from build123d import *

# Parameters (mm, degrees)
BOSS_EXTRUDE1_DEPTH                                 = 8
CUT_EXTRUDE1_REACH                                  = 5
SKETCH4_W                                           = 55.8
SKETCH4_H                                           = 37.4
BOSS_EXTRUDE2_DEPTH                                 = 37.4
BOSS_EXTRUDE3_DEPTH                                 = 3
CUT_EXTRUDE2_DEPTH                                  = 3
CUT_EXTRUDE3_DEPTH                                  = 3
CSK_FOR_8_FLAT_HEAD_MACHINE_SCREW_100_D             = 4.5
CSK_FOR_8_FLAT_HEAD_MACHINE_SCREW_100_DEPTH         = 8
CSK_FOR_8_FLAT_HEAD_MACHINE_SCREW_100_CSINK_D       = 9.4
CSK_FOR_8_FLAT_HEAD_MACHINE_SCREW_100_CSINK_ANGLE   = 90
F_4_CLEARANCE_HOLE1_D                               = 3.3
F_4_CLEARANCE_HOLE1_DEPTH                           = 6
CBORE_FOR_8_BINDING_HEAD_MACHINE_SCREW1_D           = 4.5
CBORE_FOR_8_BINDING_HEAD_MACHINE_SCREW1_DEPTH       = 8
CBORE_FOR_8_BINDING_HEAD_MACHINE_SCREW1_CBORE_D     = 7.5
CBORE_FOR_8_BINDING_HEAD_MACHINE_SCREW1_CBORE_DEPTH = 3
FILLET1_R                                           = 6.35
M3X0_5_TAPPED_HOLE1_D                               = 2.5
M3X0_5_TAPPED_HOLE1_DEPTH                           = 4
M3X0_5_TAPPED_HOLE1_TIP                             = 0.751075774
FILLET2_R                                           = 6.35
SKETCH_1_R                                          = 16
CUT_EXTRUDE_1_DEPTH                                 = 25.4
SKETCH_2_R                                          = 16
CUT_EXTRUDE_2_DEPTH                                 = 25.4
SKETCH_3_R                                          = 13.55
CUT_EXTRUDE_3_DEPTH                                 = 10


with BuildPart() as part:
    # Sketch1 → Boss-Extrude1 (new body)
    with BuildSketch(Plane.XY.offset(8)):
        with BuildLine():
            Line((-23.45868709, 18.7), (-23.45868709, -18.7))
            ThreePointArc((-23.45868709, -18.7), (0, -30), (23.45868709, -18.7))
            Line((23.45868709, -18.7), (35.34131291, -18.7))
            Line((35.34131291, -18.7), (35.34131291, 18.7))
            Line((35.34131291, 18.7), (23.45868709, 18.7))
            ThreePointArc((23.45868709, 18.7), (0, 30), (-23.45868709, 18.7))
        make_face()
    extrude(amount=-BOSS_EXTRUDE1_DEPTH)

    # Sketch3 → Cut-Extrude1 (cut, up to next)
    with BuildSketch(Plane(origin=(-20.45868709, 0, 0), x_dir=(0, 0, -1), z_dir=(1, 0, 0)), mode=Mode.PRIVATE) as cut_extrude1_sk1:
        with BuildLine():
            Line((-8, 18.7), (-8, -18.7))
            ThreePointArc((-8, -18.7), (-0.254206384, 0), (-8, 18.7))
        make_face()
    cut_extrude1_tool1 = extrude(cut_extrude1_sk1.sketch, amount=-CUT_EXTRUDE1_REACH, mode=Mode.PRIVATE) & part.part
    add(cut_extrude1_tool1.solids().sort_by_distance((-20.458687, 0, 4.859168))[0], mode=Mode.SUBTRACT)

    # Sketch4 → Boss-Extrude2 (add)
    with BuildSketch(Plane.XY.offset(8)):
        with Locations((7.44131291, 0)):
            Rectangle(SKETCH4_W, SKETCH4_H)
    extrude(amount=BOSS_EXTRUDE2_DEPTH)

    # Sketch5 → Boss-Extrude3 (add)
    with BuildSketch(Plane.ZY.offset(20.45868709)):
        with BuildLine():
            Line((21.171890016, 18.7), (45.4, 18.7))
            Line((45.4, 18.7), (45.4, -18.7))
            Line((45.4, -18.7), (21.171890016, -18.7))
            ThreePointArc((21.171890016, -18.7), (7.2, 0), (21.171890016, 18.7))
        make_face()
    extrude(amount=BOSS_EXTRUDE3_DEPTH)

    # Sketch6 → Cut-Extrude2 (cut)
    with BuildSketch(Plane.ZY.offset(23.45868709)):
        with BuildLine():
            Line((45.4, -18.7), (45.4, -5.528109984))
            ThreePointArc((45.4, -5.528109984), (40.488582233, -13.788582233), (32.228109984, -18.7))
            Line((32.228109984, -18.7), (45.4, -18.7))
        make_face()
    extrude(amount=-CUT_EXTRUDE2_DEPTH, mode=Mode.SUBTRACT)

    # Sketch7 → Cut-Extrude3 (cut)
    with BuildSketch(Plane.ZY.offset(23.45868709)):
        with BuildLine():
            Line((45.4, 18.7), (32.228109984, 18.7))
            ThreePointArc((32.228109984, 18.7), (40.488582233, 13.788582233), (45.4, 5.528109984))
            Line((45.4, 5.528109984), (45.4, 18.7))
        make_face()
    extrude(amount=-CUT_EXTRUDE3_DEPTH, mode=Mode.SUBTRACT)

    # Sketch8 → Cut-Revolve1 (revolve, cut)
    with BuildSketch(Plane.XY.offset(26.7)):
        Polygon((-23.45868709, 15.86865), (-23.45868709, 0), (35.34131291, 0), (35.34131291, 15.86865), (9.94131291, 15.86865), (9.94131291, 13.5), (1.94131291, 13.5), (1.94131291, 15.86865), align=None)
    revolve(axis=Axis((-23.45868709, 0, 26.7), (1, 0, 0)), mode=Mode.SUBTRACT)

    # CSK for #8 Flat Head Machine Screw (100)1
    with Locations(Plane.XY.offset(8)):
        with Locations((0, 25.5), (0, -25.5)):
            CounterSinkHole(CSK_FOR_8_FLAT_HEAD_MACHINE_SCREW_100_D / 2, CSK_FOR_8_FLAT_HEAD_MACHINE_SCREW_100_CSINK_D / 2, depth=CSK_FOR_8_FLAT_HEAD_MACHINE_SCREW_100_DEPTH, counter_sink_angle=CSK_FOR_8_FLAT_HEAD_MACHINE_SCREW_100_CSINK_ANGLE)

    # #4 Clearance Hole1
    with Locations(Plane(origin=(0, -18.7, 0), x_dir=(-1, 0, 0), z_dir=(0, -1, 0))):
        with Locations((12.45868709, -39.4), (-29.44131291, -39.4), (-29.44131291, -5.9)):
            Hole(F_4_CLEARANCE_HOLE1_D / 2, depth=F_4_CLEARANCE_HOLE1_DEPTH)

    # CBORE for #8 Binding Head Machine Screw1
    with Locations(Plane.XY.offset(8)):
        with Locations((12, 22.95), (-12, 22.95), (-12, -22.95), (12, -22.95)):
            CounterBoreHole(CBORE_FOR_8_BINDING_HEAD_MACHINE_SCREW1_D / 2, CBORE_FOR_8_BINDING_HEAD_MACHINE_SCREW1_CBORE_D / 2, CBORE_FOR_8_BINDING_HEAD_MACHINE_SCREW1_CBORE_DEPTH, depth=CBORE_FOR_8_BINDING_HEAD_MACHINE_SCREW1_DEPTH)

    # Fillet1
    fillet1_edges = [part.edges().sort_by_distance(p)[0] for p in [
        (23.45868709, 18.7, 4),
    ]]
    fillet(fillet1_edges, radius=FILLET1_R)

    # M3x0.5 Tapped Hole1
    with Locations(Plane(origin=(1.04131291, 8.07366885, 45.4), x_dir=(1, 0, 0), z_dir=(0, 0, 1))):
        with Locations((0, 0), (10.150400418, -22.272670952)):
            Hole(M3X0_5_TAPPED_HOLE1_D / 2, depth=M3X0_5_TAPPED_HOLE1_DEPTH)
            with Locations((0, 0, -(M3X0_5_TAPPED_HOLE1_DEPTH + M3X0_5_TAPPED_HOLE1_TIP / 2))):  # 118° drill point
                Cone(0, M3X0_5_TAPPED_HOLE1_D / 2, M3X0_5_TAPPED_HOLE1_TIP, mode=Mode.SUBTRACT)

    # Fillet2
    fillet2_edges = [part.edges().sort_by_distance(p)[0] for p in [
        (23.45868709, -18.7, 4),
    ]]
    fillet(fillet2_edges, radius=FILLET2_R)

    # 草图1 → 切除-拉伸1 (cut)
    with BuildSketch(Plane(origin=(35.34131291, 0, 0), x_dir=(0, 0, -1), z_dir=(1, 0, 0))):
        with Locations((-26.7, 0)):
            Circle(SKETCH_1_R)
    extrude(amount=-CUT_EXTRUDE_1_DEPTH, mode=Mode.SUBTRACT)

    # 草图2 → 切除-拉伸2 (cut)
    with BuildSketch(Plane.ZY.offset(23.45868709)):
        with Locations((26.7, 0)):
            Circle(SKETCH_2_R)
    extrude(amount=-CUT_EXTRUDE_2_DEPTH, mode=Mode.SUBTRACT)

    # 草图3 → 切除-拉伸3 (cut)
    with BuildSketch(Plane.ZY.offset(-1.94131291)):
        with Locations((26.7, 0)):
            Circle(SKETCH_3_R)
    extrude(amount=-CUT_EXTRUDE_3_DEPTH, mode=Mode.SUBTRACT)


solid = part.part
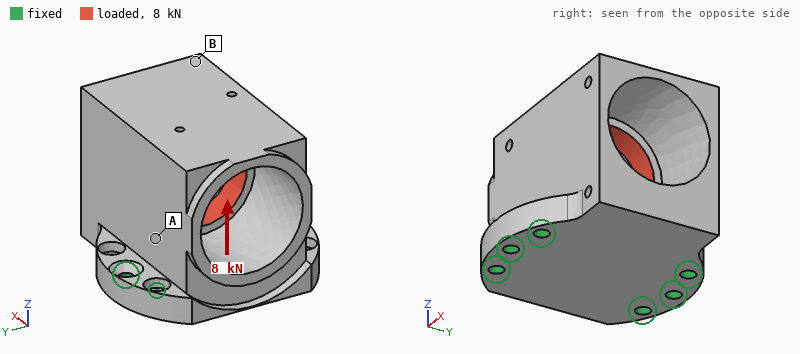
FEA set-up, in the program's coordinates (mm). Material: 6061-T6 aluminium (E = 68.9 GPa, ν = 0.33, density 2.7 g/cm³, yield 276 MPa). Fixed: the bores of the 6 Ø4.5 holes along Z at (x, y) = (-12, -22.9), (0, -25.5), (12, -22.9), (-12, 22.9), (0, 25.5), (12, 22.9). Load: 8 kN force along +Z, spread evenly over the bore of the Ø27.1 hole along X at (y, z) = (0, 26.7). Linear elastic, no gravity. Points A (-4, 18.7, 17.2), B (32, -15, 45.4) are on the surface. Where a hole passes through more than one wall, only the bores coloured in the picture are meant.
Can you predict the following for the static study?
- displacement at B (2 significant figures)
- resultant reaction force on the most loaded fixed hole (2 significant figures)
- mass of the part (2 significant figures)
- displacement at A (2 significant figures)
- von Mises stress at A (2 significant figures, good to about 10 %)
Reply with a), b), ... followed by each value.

a) 24 µm
b) 2.6 kN
c) 160 g
d) 8.8 µm
e) 24 MPa
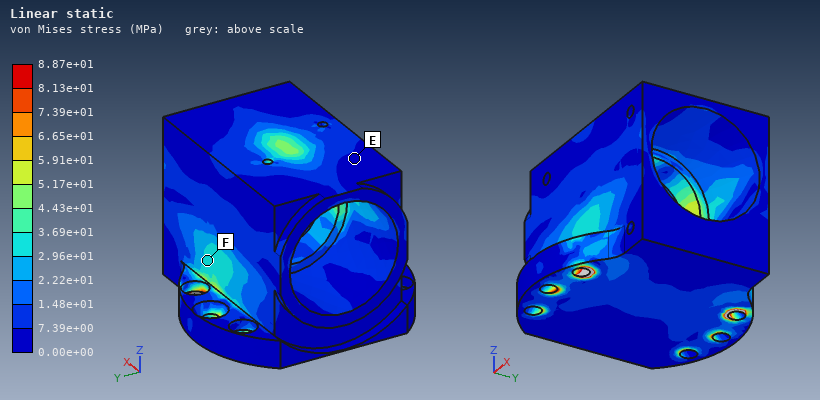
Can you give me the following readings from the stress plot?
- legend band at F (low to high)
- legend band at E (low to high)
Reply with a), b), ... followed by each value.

a) 2.96e+01 to 3.69e+01 MPa
b) 0.00e+00 to 7.39e+00 MPa
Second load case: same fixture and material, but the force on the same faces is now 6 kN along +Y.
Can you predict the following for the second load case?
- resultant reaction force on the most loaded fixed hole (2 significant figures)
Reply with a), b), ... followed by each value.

a) 2.0 kN
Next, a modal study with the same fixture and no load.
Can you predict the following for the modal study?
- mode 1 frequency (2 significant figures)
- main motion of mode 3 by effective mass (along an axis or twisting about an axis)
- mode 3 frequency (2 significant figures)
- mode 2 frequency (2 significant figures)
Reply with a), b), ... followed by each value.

a) 4800 Hz
b) twisting about Z
c) 8100 Hz
d) 4800 Hz
